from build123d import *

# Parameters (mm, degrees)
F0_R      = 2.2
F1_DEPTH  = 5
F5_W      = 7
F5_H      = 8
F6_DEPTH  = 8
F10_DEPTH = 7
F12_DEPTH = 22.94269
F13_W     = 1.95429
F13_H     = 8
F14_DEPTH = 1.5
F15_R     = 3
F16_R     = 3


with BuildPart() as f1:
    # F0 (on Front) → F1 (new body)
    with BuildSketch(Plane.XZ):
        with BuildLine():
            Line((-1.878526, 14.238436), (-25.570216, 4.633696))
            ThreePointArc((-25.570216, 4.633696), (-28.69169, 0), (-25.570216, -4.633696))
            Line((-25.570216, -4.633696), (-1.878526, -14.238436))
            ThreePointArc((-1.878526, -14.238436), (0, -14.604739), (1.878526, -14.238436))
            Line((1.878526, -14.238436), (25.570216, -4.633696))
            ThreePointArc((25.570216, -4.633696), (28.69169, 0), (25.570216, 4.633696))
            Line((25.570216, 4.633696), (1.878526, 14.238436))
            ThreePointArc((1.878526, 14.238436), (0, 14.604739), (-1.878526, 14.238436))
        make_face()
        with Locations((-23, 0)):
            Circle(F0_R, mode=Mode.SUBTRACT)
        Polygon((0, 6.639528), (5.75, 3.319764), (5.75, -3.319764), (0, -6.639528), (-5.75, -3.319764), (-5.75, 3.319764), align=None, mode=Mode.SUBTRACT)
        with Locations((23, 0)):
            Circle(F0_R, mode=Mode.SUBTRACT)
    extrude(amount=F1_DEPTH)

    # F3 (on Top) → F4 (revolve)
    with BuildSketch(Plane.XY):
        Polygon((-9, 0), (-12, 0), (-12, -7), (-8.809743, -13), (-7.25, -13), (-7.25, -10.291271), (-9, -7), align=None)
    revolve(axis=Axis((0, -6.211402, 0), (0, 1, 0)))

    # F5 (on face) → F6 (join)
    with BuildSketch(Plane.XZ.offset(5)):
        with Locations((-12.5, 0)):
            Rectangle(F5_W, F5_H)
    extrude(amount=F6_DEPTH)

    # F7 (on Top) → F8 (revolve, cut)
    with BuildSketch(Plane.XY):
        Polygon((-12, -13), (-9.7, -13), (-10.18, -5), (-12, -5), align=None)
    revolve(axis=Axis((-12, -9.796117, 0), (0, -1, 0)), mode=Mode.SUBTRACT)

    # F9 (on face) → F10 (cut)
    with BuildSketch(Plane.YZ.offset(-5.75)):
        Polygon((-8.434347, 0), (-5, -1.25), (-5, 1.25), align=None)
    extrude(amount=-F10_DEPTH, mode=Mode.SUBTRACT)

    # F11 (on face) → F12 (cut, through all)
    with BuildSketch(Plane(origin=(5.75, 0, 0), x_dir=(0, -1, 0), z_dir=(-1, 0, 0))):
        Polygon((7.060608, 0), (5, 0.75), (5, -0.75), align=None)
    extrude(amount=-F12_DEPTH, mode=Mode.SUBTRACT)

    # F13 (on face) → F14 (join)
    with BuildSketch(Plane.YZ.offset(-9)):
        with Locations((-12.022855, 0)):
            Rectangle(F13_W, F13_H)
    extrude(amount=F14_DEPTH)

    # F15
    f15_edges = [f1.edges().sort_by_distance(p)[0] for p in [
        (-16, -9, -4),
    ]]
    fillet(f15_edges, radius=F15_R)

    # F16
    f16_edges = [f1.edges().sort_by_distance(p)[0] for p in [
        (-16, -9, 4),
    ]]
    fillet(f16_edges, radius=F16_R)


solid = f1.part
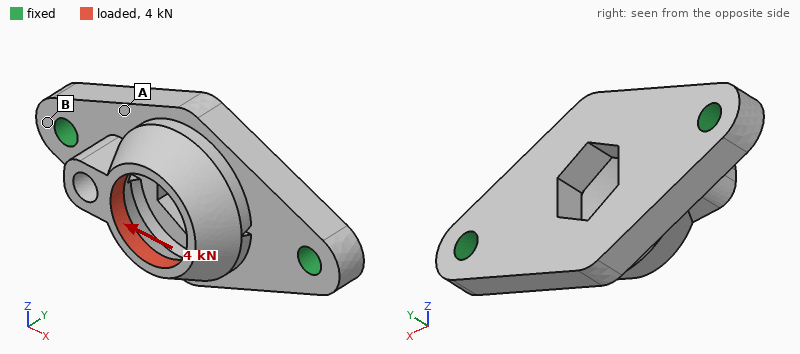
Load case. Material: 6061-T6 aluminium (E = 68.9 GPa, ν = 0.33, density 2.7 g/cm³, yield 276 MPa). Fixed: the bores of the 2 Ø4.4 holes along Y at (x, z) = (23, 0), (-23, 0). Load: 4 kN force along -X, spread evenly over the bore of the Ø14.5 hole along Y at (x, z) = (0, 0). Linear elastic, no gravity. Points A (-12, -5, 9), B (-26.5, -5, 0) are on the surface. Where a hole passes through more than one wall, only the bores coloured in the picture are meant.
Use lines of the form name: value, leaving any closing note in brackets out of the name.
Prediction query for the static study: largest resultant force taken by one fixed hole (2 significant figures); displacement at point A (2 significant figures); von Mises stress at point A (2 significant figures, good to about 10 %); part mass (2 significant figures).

largest resultant force taken by one fixed hole: 2.3 kN
displacement at point A: 10 µm
von Mises stress at point A: 43 MPa
part mass: 16 g
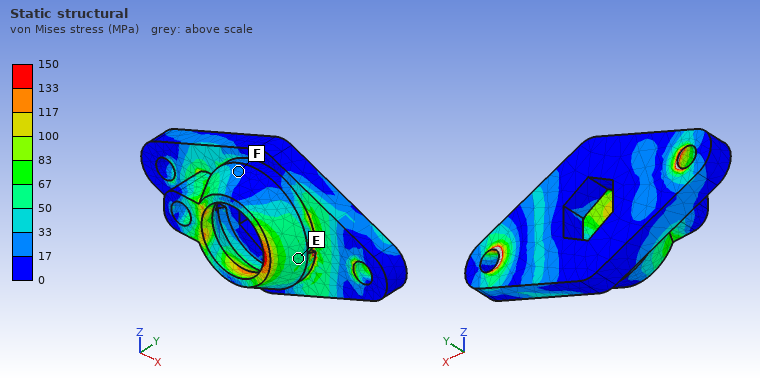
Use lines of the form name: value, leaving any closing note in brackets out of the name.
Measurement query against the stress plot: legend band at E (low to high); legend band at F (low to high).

legend band at E: 50 to 67 MPa
legend band at F: 17 to 33 MPa
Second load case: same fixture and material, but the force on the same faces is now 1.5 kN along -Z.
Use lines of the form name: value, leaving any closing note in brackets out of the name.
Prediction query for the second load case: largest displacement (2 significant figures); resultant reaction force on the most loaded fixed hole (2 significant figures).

largest displacement: 84 µm
resultant reaction force on the most loaded fixed hole: 760 N
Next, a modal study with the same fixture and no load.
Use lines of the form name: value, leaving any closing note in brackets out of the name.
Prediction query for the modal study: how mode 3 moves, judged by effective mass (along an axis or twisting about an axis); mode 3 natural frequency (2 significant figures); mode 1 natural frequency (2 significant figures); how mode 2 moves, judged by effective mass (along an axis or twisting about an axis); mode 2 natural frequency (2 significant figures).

how mode 3 moves, judged by effective mass: along Z
mode 3 natural frequency: 20 kHz
mode 1 natural frequency: 8900 Hz
how mode 2 moves, judged by effective mass: along Y
mode 2 natural frequency: 11 kHz
